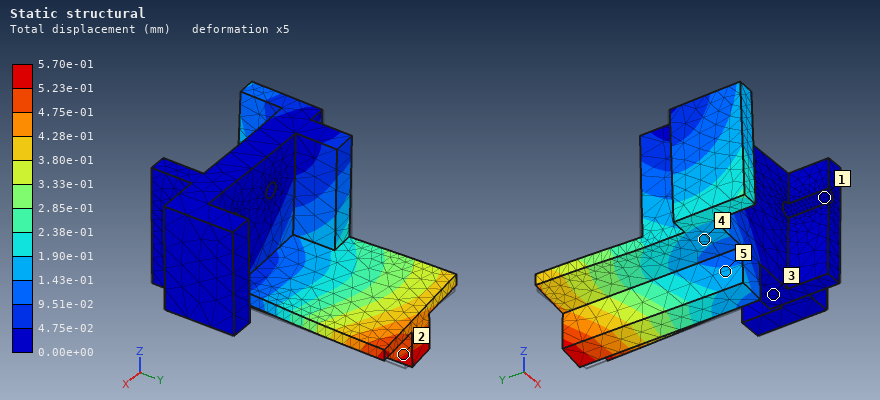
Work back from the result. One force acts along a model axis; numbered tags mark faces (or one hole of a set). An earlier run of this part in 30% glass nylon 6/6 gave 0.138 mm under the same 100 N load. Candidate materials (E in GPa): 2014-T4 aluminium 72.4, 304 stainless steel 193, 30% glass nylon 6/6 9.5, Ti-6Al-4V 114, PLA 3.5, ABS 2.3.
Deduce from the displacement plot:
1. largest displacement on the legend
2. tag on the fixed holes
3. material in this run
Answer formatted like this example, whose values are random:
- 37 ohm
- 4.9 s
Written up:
- 5.70e-01 mm
- 1
- ABS
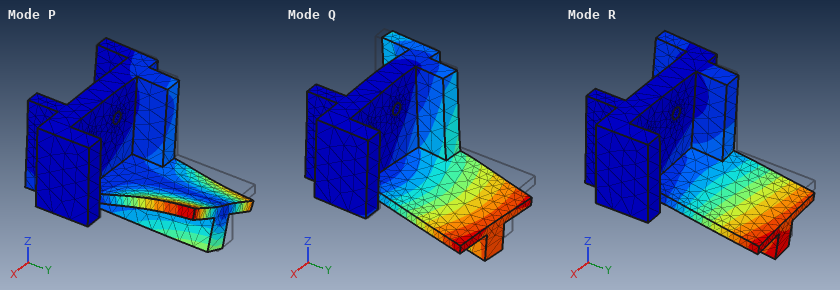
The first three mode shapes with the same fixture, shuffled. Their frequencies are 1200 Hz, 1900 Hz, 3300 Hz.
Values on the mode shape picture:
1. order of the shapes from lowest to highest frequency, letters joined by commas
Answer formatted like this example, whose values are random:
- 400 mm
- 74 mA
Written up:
- R, Q, P
